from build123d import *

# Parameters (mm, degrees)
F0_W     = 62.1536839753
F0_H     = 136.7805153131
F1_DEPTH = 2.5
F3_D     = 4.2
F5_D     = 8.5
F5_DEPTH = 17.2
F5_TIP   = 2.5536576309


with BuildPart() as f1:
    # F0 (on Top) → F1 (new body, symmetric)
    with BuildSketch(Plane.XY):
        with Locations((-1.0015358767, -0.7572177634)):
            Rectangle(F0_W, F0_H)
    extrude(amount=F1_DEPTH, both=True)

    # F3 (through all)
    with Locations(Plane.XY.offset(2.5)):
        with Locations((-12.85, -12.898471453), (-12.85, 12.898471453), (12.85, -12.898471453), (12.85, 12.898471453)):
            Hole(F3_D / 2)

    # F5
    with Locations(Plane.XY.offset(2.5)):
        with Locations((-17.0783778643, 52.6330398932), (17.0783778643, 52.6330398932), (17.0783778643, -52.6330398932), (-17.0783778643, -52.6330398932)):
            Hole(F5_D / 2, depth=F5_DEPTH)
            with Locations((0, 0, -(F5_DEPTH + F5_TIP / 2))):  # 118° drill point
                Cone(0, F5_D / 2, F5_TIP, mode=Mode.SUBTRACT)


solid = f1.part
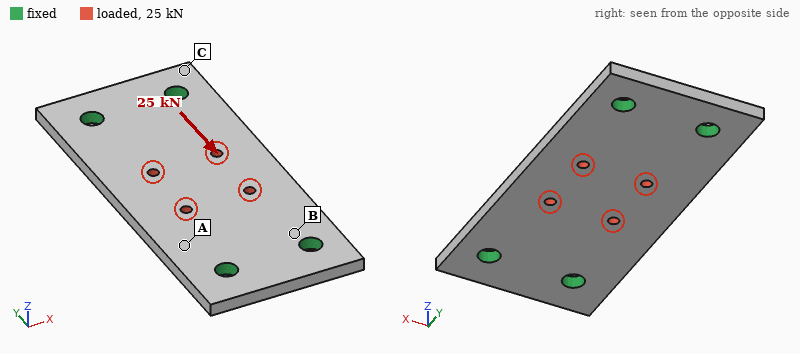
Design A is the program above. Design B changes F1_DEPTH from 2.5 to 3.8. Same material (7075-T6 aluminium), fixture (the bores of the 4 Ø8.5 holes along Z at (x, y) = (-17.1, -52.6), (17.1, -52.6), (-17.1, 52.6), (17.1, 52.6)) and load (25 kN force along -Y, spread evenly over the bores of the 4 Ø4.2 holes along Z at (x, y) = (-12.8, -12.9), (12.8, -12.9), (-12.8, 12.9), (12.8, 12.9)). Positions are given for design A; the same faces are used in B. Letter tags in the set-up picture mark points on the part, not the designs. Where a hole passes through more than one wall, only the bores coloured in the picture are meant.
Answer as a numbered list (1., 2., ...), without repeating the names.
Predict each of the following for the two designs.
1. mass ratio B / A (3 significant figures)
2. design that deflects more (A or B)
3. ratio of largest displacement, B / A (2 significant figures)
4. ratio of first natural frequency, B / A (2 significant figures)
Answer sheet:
1. 1.52
2. A
3. 0.66
4. 1.5
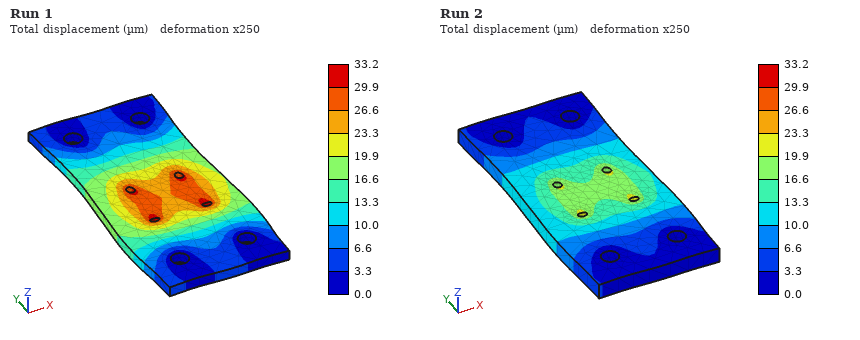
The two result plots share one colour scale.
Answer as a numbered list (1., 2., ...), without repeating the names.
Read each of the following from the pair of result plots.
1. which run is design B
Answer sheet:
1. Run 2
